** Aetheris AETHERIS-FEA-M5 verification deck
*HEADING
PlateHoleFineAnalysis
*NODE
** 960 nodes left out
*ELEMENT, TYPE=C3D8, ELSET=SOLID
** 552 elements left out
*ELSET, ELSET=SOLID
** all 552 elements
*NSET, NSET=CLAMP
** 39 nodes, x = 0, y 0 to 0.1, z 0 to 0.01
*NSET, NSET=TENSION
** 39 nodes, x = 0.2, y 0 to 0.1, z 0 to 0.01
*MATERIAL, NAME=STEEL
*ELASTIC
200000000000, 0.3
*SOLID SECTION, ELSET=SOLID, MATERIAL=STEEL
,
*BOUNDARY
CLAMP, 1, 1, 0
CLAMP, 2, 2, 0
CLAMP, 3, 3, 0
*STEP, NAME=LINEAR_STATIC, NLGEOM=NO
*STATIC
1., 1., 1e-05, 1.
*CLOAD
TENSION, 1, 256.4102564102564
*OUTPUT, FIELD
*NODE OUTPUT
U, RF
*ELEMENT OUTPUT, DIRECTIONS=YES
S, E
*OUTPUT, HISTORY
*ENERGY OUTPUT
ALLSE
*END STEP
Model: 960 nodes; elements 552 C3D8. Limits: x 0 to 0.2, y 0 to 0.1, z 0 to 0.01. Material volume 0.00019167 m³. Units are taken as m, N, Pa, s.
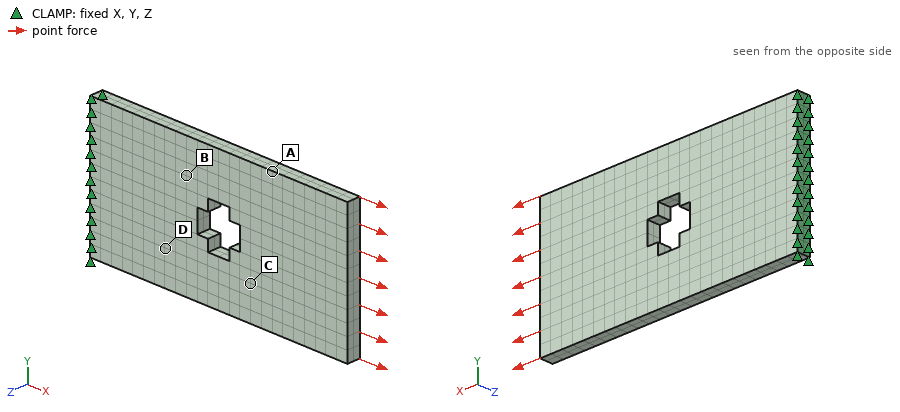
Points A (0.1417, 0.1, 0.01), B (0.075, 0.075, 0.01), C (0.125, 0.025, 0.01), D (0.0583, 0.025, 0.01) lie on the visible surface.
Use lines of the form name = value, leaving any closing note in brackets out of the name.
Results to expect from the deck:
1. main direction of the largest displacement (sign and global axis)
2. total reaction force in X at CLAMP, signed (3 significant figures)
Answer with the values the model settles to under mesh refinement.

main direction of the largest displacement = +X
total reaction force in X at CLAMP, signed = -10000 N
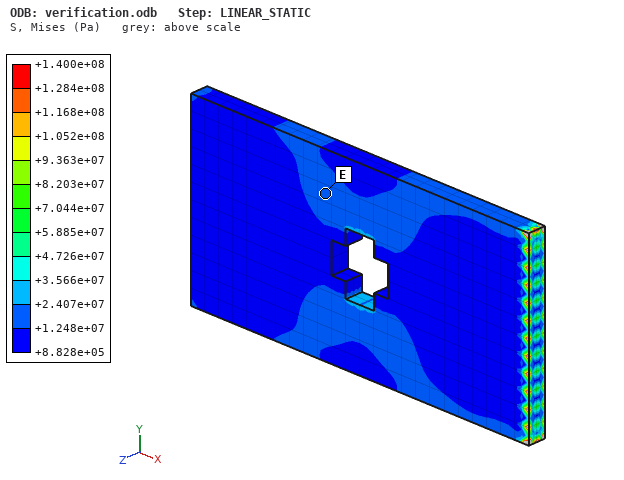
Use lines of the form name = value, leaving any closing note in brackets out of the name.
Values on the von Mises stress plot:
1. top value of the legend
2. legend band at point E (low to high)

top value of the legend = +1.400e+08 Pa
legend band at point E = +1.248e+07 to +2.407e+07 Pa
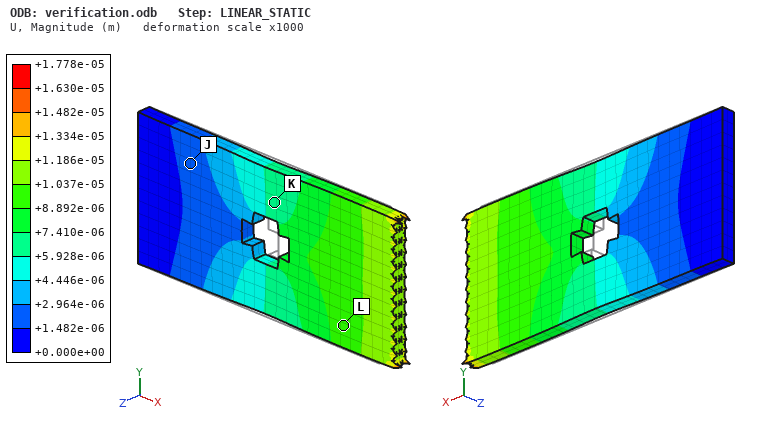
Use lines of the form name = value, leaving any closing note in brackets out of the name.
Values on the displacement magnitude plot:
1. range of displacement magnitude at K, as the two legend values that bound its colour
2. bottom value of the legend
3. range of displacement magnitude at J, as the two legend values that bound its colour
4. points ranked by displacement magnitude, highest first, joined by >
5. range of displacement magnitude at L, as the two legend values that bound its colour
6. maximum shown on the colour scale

range of displacement magnitude at K, as the two legend values that bound its colour = +5.928e-06 to +7.410e-06 m
bottom value of the legend = +0.000e+00 m
range of displacement magnitude at J, as the two legend values that bound its colour = +1.482e-06 to +2.964e-06 m
points ranked by displacement magnitude, highest first, joined by > = L > K > J
range of displacement magnitude at L, as the two legend values that bound its colour = +8.892e-06 to +1.037e-05 m
maximum shown on the colour scale = +1.778e-05 m
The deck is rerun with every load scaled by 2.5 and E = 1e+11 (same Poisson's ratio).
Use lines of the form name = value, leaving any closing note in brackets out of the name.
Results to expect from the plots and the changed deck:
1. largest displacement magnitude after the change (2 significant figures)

largest displacement magnitude after the change = 8.9e-05 m
